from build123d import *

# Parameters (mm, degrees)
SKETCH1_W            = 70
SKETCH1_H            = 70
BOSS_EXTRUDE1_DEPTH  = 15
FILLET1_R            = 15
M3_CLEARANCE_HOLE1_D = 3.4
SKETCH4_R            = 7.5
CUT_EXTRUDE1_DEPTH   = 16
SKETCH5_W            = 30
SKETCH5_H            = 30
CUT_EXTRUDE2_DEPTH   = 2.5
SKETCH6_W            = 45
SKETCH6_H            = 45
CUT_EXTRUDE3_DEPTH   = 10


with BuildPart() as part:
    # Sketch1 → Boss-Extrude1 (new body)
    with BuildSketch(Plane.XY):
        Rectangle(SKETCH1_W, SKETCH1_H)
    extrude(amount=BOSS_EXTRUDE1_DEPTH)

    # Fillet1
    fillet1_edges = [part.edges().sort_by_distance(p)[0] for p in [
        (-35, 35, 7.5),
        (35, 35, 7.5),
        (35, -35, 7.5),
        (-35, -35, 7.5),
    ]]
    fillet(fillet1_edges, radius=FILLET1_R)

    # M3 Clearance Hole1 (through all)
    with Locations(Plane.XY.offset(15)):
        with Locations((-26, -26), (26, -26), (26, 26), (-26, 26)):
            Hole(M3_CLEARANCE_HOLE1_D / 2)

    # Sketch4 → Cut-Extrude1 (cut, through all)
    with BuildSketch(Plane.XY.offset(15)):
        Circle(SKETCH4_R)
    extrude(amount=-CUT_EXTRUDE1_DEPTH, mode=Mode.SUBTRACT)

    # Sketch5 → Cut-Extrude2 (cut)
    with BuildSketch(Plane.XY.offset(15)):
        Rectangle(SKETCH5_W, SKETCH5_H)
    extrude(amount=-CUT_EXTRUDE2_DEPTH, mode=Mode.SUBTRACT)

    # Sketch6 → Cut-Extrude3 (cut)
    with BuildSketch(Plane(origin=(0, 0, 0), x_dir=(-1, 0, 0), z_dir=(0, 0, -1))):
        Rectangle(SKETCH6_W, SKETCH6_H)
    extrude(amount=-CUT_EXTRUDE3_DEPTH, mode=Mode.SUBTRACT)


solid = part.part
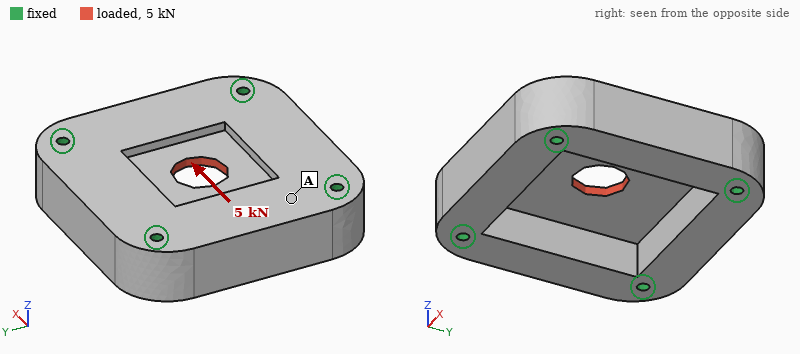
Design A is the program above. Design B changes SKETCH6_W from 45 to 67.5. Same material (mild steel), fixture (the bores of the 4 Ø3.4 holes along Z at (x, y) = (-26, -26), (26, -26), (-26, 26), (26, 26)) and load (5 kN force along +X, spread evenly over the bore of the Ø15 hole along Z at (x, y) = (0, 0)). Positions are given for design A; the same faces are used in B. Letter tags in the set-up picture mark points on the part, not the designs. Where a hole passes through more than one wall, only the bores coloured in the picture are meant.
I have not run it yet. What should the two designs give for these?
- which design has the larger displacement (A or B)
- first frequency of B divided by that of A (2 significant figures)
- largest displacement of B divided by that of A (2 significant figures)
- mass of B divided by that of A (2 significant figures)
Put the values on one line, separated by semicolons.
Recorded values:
B; 0.75; 1.2; 0.79
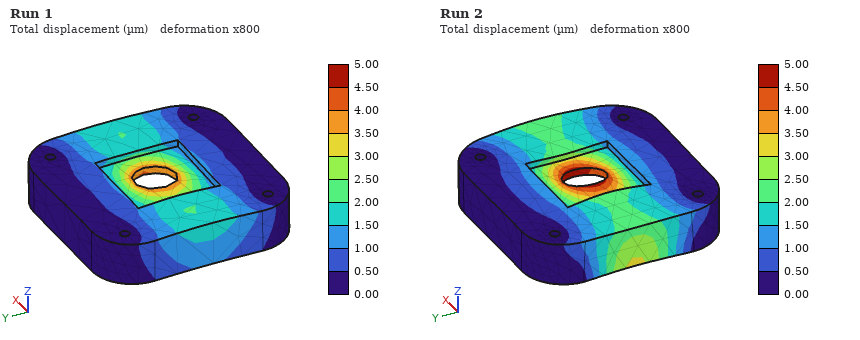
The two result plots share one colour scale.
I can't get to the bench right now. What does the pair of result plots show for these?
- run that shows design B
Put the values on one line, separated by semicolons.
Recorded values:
Run 2
